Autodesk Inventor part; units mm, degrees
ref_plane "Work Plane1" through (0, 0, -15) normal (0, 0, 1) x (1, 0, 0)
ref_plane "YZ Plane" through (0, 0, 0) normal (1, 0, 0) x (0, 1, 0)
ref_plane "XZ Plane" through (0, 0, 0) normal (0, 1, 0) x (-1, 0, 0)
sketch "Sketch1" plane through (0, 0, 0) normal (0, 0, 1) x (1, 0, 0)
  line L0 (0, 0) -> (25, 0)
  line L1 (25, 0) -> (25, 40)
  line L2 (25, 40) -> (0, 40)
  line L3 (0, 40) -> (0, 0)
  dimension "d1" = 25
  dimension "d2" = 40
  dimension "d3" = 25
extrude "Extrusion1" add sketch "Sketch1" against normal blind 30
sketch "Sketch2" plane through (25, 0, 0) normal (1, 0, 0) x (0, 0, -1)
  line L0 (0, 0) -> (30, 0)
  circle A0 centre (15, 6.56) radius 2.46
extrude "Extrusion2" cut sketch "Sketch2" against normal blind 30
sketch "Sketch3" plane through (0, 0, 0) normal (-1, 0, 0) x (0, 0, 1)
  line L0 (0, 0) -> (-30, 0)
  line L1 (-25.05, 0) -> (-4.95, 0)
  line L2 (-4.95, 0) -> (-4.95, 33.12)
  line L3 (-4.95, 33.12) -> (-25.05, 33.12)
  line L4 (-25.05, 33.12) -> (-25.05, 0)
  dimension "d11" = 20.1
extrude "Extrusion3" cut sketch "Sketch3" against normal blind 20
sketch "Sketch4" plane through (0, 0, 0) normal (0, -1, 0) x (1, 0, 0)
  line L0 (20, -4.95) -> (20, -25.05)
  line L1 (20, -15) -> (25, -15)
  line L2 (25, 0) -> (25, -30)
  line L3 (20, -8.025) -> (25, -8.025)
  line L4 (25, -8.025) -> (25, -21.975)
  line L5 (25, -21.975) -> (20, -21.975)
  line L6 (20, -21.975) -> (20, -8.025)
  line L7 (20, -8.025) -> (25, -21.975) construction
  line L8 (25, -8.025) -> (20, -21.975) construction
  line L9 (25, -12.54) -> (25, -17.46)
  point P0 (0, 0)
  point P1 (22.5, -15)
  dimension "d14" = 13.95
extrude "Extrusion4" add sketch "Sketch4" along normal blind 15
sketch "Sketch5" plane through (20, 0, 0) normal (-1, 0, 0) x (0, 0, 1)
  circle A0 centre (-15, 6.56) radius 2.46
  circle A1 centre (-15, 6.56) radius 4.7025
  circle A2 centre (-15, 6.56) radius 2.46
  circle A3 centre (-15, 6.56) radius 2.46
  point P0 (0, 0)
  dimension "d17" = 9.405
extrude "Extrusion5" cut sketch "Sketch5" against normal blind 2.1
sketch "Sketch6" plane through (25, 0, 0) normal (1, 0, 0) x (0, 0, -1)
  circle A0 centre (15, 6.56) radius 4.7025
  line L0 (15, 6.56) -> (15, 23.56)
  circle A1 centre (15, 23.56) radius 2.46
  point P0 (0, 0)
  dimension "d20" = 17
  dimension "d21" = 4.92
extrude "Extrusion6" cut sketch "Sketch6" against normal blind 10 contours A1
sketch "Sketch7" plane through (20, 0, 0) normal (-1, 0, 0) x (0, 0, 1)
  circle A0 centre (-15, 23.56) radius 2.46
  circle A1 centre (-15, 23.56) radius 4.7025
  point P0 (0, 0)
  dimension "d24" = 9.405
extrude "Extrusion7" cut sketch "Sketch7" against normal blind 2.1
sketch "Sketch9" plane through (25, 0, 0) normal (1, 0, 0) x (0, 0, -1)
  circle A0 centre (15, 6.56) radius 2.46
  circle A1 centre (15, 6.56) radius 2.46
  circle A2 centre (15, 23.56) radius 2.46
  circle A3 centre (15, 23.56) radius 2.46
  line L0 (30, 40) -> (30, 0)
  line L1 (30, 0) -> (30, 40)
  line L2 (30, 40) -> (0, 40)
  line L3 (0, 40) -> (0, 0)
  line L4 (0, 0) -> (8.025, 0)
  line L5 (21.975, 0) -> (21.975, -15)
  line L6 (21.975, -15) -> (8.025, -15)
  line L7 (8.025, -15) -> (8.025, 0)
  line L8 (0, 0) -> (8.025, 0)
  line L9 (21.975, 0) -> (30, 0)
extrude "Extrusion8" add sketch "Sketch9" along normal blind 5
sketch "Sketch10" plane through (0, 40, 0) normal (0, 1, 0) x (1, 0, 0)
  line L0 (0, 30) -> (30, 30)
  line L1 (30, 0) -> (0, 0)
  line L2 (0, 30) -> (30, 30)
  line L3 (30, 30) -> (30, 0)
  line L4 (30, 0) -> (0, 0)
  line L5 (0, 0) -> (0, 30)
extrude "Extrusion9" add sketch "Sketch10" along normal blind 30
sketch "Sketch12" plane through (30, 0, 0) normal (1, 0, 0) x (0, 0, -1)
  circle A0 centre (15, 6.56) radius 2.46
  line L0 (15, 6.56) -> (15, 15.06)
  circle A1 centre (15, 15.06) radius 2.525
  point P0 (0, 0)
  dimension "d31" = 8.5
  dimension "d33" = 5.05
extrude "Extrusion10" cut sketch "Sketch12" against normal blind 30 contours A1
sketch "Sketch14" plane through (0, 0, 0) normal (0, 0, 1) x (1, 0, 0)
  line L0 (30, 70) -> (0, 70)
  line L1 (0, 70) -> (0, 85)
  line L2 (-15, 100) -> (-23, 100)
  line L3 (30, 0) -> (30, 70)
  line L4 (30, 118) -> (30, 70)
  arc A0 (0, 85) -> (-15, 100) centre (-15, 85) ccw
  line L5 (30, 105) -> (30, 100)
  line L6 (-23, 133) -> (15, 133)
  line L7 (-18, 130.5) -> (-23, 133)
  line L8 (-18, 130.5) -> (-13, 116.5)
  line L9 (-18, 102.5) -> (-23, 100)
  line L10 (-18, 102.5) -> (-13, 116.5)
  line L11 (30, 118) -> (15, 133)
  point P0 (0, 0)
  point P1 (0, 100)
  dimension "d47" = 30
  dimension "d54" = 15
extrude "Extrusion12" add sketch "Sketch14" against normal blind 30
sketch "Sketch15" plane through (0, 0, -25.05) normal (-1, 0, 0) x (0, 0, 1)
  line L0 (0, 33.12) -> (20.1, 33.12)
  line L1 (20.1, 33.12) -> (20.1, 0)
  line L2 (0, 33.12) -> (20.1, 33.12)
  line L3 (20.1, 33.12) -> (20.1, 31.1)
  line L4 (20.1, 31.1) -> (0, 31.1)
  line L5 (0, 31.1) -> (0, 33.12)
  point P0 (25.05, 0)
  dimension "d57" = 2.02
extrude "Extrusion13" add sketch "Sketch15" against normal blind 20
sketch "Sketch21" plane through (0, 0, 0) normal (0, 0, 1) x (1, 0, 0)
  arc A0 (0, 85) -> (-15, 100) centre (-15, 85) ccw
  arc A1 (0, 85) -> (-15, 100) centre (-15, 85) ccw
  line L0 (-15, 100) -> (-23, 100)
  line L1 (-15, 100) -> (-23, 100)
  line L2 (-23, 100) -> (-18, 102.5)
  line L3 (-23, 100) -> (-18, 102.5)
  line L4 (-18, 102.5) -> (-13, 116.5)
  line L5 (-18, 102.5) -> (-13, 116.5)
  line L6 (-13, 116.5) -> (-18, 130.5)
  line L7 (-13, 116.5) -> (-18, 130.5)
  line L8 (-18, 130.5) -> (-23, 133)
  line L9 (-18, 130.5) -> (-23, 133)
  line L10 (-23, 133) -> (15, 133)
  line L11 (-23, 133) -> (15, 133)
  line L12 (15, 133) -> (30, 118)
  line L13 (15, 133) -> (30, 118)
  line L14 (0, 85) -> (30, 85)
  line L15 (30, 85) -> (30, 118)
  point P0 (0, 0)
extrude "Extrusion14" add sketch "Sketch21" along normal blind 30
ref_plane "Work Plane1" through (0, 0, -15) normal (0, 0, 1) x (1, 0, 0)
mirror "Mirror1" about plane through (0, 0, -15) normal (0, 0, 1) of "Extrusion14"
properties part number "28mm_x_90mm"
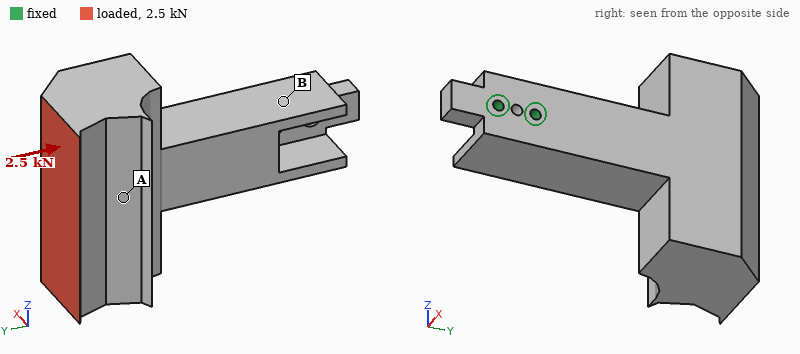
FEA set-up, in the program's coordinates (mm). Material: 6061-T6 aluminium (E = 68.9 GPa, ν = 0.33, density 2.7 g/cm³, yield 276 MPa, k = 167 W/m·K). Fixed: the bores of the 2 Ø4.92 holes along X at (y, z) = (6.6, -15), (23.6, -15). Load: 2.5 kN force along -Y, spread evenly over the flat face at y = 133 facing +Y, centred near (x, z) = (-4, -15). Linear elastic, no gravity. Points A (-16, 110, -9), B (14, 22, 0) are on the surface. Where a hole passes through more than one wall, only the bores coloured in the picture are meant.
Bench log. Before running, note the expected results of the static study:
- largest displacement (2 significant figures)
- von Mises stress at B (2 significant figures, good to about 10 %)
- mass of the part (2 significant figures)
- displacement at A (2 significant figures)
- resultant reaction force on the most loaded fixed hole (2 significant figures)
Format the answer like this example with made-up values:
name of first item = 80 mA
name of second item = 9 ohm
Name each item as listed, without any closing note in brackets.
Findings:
largest displacement = 0.25 mm
von Mises stress at B = 21 MPa
mass of the part = 640 g
displacement at A = 0.19 mm
resultant reaction force on the most loaded fixed hole = 3.4 kN
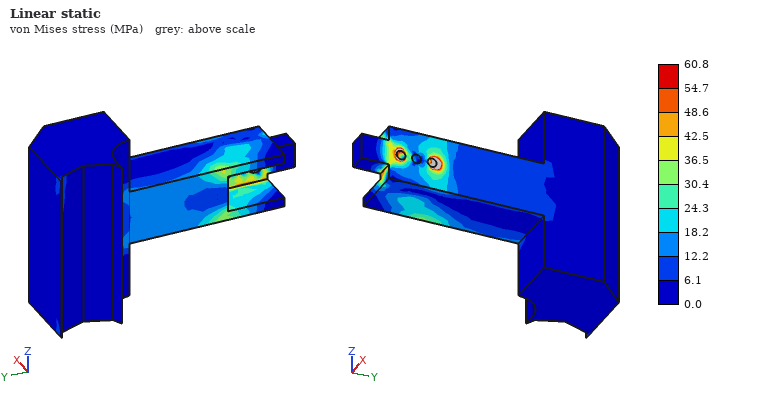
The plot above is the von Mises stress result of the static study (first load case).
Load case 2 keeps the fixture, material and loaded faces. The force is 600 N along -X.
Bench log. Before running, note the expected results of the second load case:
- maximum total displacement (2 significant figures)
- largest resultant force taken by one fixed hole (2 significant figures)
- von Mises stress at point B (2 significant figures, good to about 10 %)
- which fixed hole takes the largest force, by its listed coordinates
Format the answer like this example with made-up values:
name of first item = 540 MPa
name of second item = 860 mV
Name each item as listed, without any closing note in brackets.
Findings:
maximum total displacement = 0.23 mm
largest resultant force taken by one fixed hole = 3.2 kN
von Mises stress at point B = 18 MPa
which fixed hole takes the largest force, by its listed coordinates = (23.6, -15)
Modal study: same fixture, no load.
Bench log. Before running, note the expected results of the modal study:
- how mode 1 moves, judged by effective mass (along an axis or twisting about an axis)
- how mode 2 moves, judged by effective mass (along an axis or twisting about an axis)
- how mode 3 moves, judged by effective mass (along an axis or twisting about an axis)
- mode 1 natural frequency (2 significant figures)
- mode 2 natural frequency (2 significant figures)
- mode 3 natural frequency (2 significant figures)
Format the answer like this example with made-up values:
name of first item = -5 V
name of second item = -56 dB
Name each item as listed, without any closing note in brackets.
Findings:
how mode 1 moves, judged by effective mass = along X
how mode 2 moves, judged by effective mass = along Z
how mode 3 moves, judged by effective mass = twisting about Y
mode 1 natural frequency = 480 Hz
mode 2 natural frequency = 540 Hz
mode 3 natural frequency = 970 Hz
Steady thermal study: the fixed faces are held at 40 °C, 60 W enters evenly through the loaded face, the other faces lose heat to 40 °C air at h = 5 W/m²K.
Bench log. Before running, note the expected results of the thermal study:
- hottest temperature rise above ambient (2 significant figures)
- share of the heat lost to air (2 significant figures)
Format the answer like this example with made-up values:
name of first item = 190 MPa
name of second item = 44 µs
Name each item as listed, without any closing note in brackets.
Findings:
hottest temperature rise above ambient = 44 K
share of the heat lost to air = 7.1 %
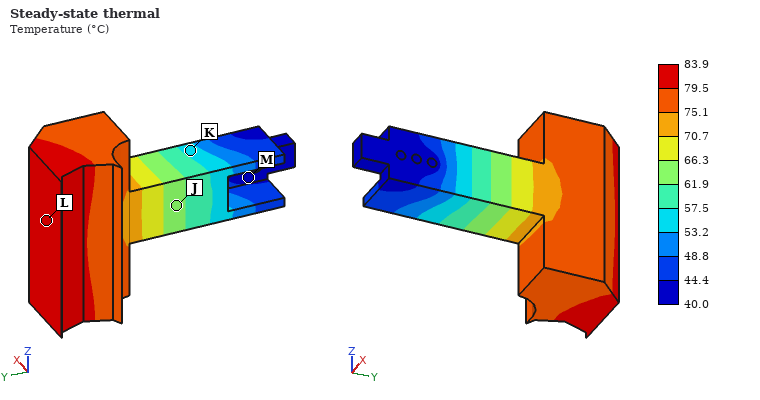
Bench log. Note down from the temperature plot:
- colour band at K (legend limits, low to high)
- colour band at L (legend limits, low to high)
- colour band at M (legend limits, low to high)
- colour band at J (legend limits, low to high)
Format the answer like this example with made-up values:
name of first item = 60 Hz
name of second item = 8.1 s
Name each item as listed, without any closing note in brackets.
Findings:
colour band at K = 53.2 to 57.5 °C
colour band at L = 79.5 to 83.9 °C
colour band at M = 40.0 to 44.4 °C
colour band at J = 61.9 to 66.3 °C
